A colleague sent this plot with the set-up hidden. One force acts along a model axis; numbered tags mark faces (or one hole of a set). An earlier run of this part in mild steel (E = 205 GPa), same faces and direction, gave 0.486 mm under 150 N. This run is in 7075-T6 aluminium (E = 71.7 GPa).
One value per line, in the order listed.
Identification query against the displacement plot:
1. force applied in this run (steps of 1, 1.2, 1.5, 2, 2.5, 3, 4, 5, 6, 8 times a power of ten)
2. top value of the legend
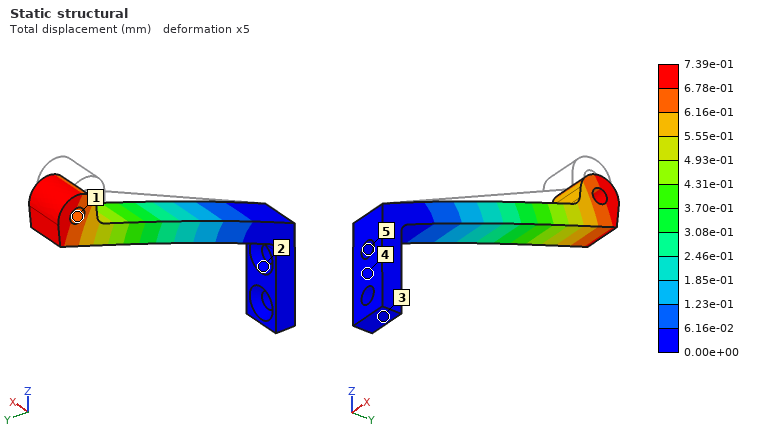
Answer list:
80 N
7.39e-01 mm
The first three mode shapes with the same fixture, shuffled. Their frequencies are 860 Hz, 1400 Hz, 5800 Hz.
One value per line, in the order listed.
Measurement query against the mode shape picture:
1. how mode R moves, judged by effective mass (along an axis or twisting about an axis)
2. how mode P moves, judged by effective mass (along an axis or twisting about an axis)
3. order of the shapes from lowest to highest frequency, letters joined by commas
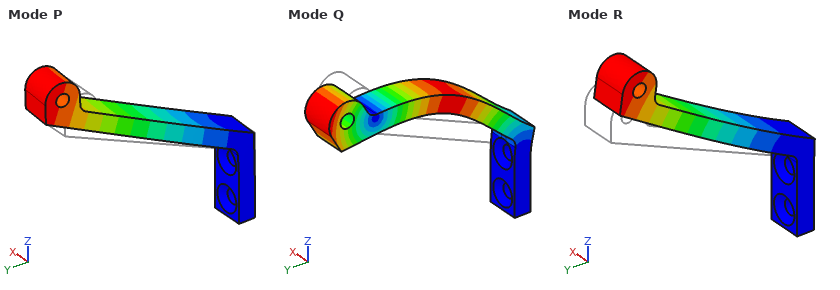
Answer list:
along Z
along X
R, P, Q
